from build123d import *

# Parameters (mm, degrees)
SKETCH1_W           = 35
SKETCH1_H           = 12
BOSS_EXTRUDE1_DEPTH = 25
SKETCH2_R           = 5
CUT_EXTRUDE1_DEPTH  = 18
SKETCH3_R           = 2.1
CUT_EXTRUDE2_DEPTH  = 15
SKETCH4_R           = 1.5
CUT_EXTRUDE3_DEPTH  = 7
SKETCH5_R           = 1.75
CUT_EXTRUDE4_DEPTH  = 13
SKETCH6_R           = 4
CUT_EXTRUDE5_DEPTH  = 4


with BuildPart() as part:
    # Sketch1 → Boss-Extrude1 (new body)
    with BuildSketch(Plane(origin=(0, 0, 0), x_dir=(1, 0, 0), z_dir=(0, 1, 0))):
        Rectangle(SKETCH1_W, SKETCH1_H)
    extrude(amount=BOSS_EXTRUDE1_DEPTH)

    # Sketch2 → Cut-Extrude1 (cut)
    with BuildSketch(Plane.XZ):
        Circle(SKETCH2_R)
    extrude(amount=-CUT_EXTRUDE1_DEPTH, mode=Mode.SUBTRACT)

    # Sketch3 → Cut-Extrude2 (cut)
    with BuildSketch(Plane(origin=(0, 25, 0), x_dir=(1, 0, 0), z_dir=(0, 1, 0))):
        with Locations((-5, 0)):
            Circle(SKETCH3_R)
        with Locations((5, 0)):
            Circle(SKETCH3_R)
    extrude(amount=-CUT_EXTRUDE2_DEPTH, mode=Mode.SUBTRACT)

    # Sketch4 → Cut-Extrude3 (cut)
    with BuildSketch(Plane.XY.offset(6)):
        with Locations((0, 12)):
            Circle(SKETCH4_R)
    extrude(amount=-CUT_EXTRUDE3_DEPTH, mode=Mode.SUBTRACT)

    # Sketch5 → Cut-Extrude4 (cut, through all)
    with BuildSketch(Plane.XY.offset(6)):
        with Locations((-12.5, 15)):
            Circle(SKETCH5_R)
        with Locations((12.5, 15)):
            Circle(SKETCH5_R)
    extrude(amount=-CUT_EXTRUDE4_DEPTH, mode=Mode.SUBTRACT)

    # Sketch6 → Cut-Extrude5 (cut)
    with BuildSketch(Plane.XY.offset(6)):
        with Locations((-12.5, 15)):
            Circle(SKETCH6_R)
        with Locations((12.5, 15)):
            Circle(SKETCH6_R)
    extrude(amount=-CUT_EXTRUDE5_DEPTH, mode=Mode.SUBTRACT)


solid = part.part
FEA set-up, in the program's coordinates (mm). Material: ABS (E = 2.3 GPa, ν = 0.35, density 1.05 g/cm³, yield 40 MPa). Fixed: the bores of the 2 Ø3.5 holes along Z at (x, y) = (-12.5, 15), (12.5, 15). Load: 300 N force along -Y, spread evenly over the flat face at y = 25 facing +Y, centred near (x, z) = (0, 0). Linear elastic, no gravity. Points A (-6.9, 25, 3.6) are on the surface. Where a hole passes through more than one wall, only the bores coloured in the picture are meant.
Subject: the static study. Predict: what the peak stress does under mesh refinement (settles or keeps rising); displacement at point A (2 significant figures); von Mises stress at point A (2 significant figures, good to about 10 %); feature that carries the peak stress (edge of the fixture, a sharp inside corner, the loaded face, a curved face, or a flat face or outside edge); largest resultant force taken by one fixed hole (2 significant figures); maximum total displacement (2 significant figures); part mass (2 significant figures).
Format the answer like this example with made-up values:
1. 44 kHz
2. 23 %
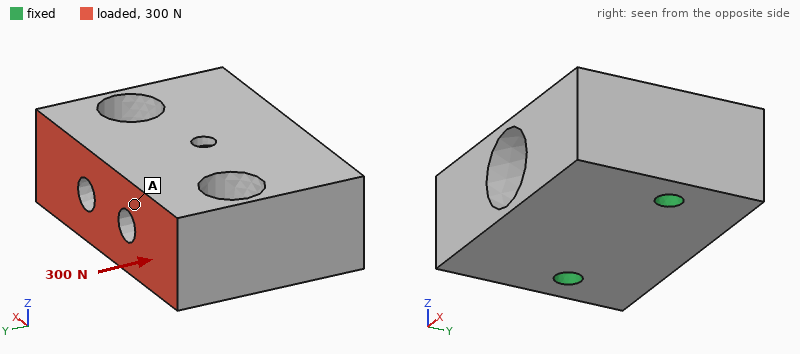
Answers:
1. keeps rising
2. 15 µm
3. 0.70 MPa
4. edge of the fixture
5. 150 N
6. 19 µm
7. 8.6 g
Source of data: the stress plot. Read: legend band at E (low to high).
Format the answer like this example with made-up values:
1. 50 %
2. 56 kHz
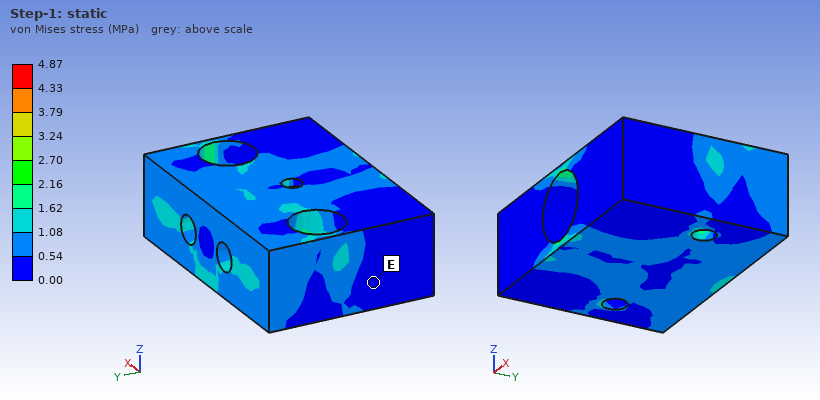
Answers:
1. 0.00 to 0.54 MPa
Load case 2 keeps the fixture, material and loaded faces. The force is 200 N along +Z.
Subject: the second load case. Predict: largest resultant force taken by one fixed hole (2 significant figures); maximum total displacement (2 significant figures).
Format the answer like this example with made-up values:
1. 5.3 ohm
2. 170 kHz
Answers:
1. 100 N
2. 49 µm
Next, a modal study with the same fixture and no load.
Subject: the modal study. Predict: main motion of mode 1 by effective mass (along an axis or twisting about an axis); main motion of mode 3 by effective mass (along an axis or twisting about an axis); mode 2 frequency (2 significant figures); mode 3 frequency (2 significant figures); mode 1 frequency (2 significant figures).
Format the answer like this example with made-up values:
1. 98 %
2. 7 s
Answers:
1. along Z
2. along X
3. 7600 Hz
4. 9300 Hz
5. 5400 Hz
